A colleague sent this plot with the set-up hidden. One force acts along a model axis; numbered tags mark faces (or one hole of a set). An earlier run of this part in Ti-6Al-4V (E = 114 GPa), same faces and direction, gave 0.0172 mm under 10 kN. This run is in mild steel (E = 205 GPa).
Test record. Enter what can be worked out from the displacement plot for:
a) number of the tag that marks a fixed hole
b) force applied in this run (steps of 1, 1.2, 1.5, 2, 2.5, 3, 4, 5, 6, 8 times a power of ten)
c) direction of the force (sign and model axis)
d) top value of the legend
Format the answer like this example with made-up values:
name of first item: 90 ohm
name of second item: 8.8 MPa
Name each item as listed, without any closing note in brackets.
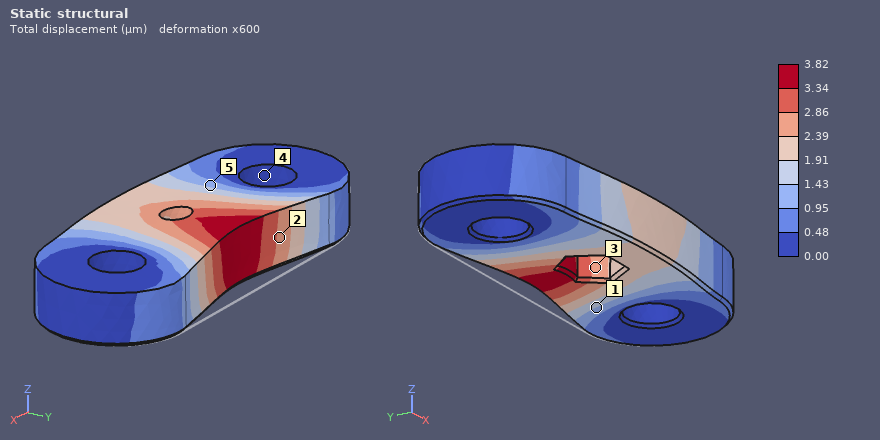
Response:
number of the tag that marks a fixed hole: 4
force applied in this run: 4 kN
direction of the force: -Y
top value of the legend: 3.82 µm
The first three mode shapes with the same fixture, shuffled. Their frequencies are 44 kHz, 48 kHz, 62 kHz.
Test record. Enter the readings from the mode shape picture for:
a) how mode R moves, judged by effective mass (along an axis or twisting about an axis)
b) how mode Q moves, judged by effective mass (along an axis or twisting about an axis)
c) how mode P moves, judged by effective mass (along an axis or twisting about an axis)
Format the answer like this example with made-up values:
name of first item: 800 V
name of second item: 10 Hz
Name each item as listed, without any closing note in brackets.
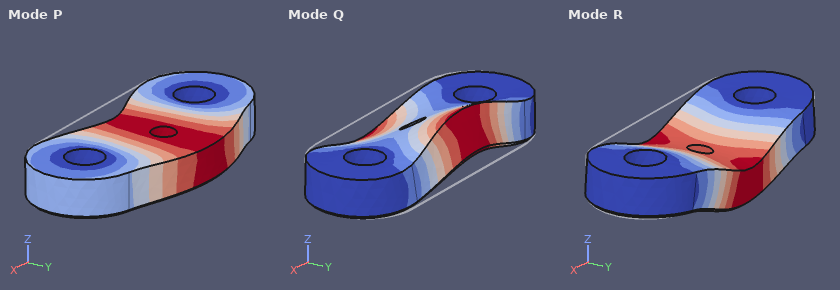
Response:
how mode R moves, judged by effective mass: along Z
how mode Q moves, judged by effective mass: twisting about X
how mode P moves, judged by effective mass: along Y
